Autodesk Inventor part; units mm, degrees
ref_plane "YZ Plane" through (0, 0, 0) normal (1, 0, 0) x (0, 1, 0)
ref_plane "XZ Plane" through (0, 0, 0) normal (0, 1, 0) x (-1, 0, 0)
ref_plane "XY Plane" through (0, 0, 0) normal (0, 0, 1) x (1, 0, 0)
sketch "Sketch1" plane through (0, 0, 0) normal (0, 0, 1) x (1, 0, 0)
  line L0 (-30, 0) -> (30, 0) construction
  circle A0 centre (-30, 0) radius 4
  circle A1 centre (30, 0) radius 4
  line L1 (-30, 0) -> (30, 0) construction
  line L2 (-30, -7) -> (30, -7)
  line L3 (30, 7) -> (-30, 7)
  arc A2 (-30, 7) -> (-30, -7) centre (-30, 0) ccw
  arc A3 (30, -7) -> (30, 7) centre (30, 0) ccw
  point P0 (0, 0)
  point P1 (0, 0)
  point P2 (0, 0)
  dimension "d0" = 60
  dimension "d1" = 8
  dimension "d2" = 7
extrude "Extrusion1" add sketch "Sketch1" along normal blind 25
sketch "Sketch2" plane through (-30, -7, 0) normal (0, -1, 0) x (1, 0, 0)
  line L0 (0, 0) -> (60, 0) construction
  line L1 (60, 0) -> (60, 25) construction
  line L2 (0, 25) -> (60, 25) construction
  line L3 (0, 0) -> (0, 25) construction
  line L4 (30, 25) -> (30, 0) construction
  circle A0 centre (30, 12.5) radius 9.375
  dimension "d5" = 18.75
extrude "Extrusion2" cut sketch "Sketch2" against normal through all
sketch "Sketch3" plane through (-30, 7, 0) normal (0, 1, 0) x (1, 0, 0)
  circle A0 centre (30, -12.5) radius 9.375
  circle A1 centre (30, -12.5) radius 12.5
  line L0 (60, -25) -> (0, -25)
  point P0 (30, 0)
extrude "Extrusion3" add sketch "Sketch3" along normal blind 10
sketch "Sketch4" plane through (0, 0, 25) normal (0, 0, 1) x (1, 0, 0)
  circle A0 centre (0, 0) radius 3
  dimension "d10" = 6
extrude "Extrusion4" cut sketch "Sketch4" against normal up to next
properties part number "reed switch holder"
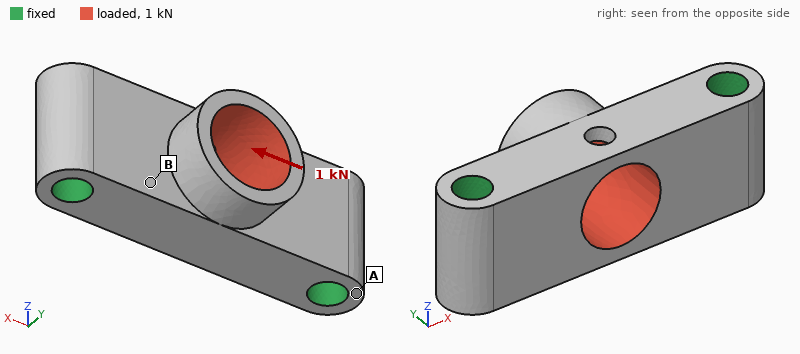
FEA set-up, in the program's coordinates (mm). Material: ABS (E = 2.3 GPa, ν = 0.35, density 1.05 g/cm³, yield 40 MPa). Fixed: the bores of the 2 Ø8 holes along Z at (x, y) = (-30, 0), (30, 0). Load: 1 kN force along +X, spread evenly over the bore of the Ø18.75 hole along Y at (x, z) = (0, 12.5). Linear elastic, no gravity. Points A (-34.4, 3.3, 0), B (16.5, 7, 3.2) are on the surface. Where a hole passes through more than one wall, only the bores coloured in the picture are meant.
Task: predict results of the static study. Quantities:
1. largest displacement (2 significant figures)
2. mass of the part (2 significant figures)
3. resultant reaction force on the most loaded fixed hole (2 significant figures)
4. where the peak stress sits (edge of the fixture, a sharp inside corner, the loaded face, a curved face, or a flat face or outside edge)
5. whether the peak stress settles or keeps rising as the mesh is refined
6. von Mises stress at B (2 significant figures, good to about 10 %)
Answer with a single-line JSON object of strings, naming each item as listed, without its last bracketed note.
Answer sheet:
{"largest displacement": "66 µm", "mass of the part": "22 g", "resultant reaction force on the most loaded fixed hole": "510 N", "where the peak stress sits": "a sharp inside corner", "whether the peak stress settles or keeps rising as the mesh is refined": "keeps rising", "von Mises stress at B": "2.3 MPa"}
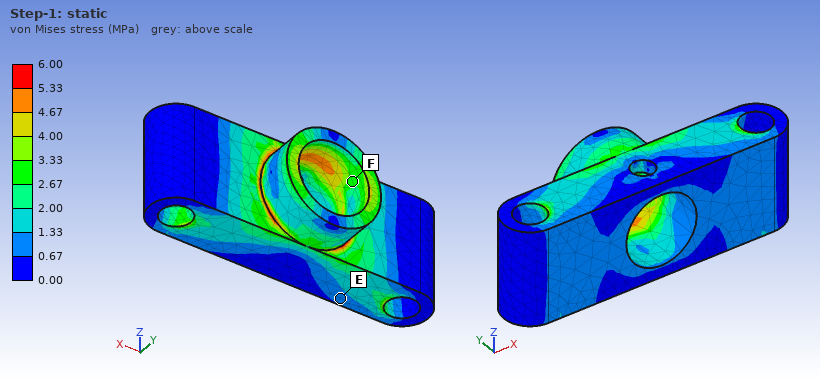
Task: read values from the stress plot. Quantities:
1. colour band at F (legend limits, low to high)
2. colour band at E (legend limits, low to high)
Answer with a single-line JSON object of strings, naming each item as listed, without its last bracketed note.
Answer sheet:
{"colour band at F": "2.67 to 3.33 MPa", "colour band at E": "0.67 to 1.33 MPa"}
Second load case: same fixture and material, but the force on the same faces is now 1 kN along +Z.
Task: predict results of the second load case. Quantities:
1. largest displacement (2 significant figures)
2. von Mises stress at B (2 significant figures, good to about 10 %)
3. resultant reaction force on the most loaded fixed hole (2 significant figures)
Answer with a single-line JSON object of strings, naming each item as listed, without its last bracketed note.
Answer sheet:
{"largest displacement": "0.18 mm", "von Mises stress at B": "3.9 MPa", "resultant reaction force on the most loaded fixed hole": "500 N"}
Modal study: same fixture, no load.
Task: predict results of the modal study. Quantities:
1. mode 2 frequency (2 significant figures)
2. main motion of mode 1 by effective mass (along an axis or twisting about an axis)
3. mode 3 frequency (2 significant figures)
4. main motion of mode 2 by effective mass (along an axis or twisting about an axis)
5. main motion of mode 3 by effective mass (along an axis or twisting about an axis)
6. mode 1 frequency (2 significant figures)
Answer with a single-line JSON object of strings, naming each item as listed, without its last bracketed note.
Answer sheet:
{"mode 2 frequency": "5200 Hz", "main motion of mode 1 by effective mass": "along Y", "mode 3 frequency": "7700 Hz", "main motion of mode 2 by effective mass": "along Z", "main motion of mode 3 by effective mass": "along Z", "mode 1 frequency": "4800 Hz"}
